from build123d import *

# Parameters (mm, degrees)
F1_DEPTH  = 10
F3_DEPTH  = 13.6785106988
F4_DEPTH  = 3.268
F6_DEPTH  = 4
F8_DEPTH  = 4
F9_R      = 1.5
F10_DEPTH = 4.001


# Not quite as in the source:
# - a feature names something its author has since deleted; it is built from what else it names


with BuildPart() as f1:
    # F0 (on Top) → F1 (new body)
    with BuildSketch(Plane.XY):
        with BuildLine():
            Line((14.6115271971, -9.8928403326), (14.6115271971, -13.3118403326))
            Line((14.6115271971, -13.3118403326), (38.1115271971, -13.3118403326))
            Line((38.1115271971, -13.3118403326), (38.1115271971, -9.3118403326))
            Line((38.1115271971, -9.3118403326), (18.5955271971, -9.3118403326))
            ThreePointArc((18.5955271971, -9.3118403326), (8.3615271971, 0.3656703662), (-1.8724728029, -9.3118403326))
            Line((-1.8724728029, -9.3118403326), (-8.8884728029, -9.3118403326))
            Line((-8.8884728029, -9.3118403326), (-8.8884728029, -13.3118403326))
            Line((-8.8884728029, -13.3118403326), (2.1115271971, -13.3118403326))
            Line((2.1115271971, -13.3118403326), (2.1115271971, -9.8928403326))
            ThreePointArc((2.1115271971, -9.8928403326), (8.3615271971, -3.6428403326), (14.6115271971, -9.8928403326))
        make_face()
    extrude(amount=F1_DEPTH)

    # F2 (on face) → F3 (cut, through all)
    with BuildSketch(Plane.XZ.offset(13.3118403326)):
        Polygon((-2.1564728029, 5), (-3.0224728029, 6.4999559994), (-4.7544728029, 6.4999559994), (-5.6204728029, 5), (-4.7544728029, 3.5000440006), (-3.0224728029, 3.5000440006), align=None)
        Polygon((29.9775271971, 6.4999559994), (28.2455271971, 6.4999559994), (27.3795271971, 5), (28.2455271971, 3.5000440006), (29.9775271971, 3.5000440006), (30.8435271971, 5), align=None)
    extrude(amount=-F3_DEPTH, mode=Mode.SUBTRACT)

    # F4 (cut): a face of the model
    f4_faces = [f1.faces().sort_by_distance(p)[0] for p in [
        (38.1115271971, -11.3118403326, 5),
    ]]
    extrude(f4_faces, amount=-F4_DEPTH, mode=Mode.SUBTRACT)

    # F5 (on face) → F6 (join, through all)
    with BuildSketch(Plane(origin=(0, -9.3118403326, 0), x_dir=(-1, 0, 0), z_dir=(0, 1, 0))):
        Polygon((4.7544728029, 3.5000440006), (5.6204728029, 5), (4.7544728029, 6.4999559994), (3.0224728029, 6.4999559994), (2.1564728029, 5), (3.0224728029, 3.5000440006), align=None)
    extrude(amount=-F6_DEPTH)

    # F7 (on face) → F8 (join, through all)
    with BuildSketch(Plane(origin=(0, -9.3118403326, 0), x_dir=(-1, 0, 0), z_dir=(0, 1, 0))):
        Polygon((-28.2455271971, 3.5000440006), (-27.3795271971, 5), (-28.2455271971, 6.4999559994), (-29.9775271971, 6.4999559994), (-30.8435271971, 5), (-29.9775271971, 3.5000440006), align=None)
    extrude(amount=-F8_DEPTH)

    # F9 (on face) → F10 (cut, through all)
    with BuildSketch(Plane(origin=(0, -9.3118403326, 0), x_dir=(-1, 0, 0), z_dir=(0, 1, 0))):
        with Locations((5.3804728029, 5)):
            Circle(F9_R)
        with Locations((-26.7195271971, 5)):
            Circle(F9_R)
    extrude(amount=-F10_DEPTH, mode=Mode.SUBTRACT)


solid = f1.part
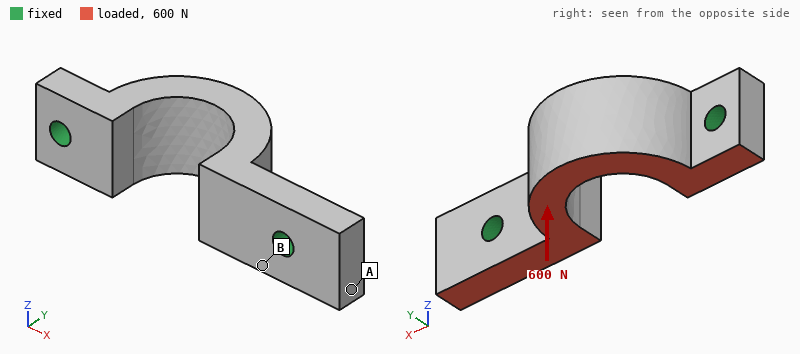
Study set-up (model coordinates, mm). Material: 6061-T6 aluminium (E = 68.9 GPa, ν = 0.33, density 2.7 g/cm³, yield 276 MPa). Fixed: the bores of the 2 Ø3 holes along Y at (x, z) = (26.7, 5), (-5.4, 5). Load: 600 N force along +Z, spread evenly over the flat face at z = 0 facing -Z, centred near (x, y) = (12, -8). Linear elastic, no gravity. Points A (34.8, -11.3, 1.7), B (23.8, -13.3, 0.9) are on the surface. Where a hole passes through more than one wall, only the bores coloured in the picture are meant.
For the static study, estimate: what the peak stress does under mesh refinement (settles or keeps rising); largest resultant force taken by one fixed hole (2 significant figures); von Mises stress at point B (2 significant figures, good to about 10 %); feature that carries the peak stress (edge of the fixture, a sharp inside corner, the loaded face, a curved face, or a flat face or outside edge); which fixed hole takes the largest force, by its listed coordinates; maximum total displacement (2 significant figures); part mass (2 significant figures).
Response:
keeps rising
320 N
18 MPa
edge of the fixture
(26.7, 5)
23 µm
5.9 g
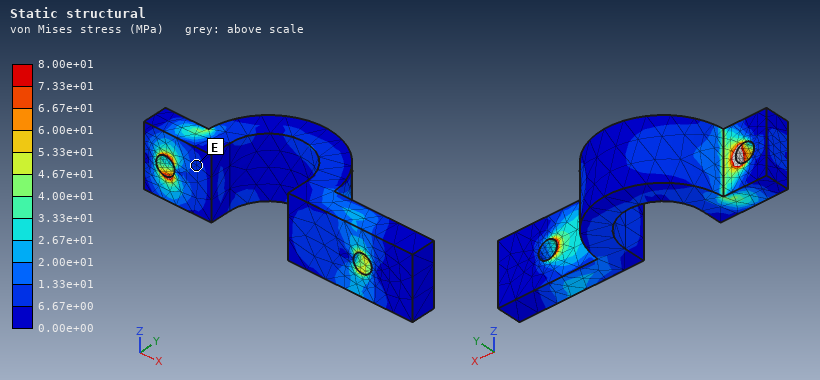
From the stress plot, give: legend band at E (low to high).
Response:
6.67e+00 to 1.33e+01 MPa
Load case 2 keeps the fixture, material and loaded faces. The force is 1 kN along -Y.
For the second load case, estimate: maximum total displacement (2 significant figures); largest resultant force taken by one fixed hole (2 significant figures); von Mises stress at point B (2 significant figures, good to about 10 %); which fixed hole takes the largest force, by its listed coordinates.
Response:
37 µm
580 N
43 MPa
(26.7, 5)
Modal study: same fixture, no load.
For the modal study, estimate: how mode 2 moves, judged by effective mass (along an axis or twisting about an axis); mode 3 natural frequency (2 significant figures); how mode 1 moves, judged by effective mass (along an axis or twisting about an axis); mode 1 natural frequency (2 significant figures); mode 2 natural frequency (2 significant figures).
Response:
along Y
29 kHz
along Z
12 kHz
21 kHz
